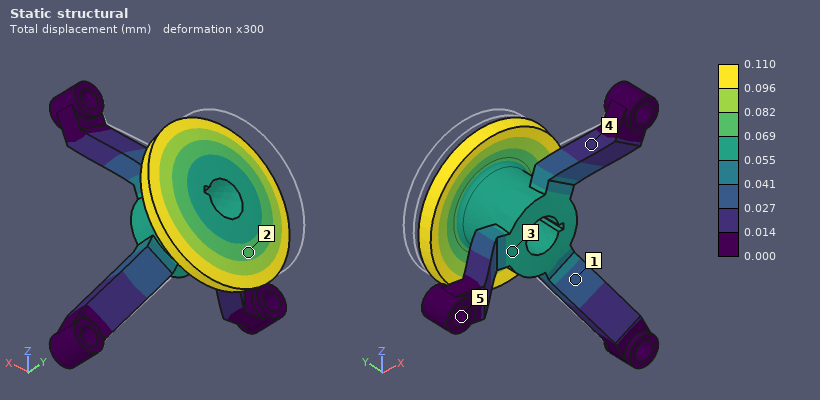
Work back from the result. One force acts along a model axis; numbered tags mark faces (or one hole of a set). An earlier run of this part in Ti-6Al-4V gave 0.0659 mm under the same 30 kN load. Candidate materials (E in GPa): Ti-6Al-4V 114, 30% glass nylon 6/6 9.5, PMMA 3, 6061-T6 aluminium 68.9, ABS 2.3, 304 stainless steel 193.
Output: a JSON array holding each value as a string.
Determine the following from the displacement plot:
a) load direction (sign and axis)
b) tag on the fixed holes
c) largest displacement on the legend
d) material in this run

["-Y", "5", "0.110 mm", "6061-T6 aluminium"]
